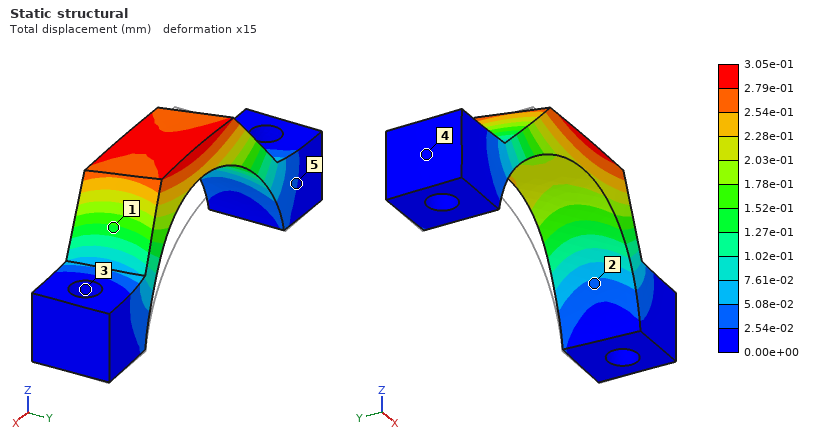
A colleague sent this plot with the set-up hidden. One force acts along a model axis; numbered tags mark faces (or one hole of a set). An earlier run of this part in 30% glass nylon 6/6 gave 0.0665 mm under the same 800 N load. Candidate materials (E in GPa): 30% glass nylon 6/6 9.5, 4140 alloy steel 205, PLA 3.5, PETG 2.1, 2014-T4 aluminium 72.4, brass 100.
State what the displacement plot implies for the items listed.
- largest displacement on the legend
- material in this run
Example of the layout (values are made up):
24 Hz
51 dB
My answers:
3.05e-01 mm
PETG
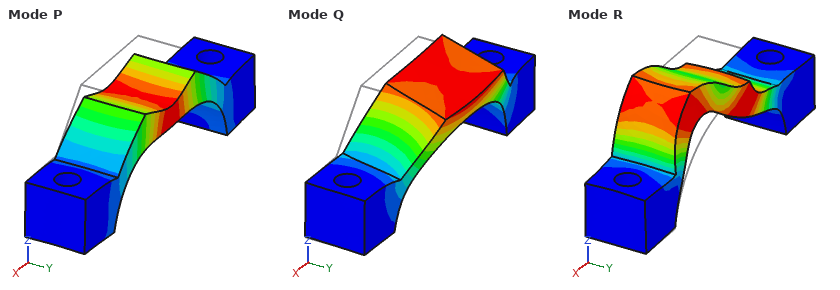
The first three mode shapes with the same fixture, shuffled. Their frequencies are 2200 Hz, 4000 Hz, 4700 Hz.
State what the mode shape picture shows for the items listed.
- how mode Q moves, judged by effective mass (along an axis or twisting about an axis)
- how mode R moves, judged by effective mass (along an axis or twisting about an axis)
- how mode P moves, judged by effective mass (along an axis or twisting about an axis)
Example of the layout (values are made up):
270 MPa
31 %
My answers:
along Y
along X
along Z
